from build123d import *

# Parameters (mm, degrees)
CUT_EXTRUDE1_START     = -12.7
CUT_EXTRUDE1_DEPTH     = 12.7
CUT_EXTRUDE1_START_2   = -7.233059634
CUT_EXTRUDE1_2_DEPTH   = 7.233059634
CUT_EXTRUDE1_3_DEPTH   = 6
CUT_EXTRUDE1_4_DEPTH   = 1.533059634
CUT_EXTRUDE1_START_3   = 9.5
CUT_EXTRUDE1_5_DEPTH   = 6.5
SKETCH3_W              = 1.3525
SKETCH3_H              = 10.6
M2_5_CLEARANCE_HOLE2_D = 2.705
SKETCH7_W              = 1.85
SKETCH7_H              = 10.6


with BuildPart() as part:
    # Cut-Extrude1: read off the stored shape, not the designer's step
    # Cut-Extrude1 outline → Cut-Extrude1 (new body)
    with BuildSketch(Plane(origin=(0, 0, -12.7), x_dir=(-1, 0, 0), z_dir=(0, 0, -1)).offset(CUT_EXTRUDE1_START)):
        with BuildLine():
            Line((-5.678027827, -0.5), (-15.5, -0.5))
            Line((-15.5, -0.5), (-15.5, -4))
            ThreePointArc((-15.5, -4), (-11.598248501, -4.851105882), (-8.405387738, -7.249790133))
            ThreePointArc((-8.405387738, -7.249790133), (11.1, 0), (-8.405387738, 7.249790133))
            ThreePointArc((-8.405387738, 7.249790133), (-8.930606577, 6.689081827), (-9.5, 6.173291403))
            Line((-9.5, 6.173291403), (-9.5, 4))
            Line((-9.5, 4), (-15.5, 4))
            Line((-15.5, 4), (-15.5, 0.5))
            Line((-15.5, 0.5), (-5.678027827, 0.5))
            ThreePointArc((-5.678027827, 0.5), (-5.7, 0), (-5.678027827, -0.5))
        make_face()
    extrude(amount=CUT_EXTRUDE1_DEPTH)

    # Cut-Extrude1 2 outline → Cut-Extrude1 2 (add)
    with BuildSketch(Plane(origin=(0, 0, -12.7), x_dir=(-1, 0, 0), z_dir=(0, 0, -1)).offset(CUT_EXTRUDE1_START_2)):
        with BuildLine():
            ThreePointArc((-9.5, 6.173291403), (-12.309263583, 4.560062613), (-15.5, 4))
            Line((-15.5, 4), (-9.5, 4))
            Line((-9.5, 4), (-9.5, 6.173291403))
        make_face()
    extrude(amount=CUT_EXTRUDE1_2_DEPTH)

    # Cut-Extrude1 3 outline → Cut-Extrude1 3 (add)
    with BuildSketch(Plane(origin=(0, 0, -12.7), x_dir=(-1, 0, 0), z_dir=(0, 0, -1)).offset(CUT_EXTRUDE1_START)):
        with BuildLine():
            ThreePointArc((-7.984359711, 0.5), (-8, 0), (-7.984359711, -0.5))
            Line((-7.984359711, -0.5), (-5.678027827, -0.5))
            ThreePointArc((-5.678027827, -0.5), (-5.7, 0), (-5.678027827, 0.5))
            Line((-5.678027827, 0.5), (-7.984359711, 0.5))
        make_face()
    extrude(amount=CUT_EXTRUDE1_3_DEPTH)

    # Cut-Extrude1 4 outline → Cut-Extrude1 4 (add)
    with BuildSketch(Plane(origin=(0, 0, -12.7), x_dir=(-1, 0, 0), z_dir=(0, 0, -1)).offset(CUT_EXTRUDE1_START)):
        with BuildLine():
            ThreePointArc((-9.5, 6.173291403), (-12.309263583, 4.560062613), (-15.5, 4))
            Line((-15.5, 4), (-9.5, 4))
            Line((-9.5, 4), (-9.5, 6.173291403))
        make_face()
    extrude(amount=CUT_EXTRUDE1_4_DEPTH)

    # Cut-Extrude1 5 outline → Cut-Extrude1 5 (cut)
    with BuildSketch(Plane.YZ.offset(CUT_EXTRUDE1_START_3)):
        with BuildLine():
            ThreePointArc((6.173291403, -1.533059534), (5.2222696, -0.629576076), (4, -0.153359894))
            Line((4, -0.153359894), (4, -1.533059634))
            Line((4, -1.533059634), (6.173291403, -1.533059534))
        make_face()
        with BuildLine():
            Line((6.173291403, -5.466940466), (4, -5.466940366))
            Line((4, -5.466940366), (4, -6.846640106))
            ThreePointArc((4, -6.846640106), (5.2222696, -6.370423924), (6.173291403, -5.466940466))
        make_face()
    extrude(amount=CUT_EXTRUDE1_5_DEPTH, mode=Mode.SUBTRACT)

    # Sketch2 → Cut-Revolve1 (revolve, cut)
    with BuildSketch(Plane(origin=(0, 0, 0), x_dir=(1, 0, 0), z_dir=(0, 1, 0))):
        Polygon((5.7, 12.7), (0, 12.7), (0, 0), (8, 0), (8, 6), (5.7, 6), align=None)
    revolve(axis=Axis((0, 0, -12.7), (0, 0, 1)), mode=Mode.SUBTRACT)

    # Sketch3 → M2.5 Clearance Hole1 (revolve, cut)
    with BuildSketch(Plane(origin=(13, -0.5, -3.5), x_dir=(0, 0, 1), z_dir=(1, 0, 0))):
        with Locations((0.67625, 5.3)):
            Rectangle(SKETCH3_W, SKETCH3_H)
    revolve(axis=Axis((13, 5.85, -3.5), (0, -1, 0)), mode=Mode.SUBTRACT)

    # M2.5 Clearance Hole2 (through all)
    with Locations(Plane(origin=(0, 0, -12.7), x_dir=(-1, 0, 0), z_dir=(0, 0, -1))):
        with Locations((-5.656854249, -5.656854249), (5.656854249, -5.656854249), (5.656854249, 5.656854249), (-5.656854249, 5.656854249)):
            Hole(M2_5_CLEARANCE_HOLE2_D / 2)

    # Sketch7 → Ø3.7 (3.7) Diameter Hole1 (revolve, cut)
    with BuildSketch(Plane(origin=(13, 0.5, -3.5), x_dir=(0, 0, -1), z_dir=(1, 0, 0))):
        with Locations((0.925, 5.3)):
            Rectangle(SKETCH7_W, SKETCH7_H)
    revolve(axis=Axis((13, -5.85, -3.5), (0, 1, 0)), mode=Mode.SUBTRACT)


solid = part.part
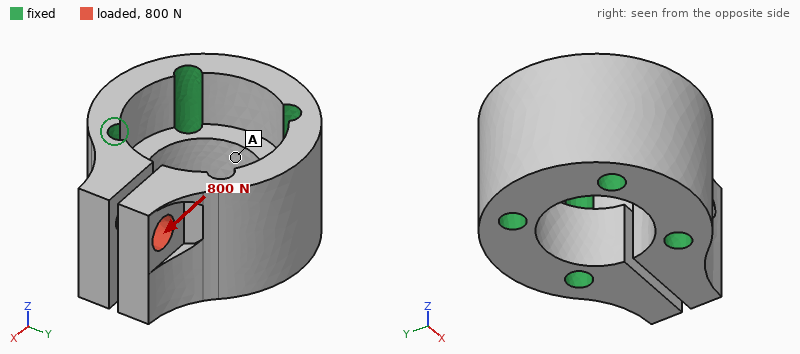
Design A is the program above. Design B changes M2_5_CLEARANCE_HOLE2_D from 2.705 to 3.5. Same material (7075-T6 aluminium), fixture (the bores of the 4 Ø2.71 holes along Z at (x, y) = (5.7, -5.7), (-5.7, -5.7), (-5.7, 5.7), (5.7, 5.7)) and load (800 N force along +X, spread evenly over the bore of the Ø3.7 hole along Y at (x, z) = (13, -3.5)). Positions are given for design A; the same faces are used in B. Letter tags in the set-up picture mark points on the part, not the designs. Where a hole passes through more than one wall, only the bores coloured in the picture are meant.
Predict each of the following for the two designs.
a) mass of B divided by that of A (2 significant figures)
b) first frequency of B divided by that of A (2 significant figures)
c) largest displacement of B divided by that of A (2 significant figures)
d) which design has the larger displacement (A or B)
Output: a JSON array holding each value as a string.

["0.95", "1.1", "0.83", "A"]
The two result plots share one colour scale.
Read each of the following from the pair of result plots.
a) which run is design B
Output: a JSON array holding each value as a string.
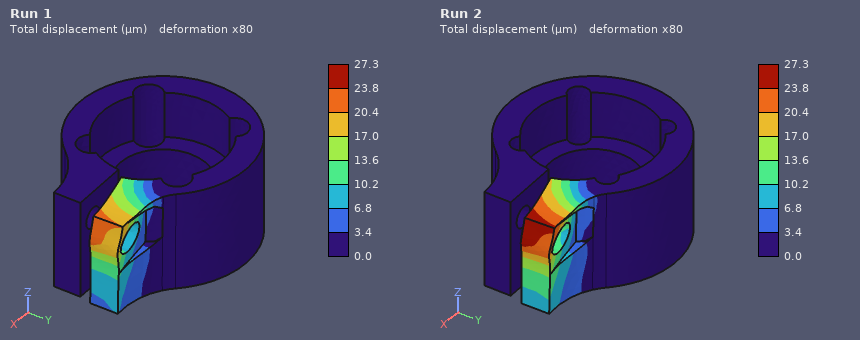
["Run 1"]
